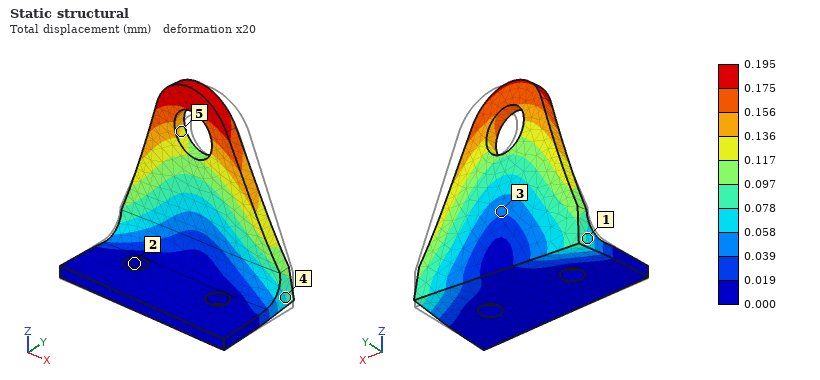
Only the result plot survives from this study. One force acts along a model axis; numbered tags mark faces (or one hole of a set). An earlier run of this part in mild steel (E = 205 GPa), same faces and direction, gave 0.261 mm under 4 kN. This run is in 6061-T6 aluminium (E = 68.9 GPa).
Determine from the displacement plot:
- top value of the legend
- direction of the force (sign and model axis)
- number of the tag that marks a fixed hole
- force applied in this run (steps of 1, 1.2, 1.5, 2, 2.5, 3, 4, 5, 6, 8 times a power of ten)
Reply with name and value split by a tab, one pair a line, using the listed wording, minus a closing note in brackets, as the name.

top value of the legend	0.195 mm
direction of the force	-X
number of the tag that marks a fixed hole	2
force applied in this run	1 kN
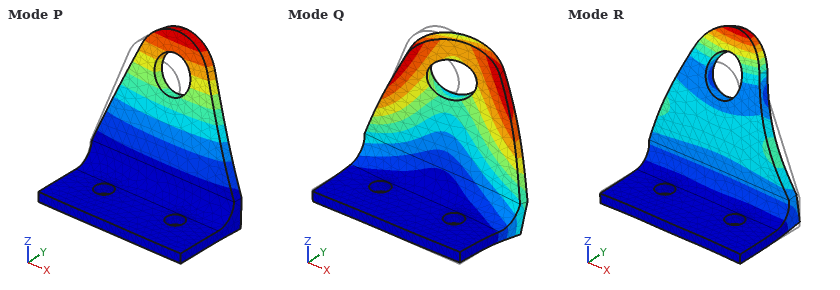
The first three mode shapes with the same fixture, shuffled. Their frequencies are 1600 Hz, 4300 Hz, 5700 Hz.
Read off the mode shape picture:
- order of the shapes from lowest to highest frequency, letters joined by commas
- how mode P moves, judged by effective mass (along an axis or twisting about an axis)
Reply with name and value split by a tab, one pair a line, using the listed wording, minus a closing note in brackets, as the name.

order of the shapes from lowest to highest frequency, letters joined by commas	P, Q, R
how mode P moves, judged by effective mass	along Y
